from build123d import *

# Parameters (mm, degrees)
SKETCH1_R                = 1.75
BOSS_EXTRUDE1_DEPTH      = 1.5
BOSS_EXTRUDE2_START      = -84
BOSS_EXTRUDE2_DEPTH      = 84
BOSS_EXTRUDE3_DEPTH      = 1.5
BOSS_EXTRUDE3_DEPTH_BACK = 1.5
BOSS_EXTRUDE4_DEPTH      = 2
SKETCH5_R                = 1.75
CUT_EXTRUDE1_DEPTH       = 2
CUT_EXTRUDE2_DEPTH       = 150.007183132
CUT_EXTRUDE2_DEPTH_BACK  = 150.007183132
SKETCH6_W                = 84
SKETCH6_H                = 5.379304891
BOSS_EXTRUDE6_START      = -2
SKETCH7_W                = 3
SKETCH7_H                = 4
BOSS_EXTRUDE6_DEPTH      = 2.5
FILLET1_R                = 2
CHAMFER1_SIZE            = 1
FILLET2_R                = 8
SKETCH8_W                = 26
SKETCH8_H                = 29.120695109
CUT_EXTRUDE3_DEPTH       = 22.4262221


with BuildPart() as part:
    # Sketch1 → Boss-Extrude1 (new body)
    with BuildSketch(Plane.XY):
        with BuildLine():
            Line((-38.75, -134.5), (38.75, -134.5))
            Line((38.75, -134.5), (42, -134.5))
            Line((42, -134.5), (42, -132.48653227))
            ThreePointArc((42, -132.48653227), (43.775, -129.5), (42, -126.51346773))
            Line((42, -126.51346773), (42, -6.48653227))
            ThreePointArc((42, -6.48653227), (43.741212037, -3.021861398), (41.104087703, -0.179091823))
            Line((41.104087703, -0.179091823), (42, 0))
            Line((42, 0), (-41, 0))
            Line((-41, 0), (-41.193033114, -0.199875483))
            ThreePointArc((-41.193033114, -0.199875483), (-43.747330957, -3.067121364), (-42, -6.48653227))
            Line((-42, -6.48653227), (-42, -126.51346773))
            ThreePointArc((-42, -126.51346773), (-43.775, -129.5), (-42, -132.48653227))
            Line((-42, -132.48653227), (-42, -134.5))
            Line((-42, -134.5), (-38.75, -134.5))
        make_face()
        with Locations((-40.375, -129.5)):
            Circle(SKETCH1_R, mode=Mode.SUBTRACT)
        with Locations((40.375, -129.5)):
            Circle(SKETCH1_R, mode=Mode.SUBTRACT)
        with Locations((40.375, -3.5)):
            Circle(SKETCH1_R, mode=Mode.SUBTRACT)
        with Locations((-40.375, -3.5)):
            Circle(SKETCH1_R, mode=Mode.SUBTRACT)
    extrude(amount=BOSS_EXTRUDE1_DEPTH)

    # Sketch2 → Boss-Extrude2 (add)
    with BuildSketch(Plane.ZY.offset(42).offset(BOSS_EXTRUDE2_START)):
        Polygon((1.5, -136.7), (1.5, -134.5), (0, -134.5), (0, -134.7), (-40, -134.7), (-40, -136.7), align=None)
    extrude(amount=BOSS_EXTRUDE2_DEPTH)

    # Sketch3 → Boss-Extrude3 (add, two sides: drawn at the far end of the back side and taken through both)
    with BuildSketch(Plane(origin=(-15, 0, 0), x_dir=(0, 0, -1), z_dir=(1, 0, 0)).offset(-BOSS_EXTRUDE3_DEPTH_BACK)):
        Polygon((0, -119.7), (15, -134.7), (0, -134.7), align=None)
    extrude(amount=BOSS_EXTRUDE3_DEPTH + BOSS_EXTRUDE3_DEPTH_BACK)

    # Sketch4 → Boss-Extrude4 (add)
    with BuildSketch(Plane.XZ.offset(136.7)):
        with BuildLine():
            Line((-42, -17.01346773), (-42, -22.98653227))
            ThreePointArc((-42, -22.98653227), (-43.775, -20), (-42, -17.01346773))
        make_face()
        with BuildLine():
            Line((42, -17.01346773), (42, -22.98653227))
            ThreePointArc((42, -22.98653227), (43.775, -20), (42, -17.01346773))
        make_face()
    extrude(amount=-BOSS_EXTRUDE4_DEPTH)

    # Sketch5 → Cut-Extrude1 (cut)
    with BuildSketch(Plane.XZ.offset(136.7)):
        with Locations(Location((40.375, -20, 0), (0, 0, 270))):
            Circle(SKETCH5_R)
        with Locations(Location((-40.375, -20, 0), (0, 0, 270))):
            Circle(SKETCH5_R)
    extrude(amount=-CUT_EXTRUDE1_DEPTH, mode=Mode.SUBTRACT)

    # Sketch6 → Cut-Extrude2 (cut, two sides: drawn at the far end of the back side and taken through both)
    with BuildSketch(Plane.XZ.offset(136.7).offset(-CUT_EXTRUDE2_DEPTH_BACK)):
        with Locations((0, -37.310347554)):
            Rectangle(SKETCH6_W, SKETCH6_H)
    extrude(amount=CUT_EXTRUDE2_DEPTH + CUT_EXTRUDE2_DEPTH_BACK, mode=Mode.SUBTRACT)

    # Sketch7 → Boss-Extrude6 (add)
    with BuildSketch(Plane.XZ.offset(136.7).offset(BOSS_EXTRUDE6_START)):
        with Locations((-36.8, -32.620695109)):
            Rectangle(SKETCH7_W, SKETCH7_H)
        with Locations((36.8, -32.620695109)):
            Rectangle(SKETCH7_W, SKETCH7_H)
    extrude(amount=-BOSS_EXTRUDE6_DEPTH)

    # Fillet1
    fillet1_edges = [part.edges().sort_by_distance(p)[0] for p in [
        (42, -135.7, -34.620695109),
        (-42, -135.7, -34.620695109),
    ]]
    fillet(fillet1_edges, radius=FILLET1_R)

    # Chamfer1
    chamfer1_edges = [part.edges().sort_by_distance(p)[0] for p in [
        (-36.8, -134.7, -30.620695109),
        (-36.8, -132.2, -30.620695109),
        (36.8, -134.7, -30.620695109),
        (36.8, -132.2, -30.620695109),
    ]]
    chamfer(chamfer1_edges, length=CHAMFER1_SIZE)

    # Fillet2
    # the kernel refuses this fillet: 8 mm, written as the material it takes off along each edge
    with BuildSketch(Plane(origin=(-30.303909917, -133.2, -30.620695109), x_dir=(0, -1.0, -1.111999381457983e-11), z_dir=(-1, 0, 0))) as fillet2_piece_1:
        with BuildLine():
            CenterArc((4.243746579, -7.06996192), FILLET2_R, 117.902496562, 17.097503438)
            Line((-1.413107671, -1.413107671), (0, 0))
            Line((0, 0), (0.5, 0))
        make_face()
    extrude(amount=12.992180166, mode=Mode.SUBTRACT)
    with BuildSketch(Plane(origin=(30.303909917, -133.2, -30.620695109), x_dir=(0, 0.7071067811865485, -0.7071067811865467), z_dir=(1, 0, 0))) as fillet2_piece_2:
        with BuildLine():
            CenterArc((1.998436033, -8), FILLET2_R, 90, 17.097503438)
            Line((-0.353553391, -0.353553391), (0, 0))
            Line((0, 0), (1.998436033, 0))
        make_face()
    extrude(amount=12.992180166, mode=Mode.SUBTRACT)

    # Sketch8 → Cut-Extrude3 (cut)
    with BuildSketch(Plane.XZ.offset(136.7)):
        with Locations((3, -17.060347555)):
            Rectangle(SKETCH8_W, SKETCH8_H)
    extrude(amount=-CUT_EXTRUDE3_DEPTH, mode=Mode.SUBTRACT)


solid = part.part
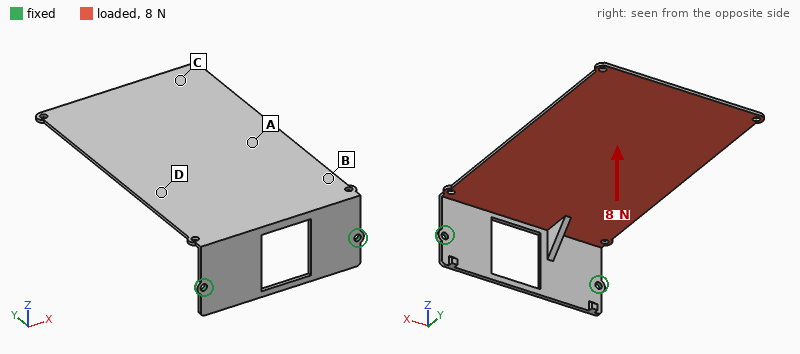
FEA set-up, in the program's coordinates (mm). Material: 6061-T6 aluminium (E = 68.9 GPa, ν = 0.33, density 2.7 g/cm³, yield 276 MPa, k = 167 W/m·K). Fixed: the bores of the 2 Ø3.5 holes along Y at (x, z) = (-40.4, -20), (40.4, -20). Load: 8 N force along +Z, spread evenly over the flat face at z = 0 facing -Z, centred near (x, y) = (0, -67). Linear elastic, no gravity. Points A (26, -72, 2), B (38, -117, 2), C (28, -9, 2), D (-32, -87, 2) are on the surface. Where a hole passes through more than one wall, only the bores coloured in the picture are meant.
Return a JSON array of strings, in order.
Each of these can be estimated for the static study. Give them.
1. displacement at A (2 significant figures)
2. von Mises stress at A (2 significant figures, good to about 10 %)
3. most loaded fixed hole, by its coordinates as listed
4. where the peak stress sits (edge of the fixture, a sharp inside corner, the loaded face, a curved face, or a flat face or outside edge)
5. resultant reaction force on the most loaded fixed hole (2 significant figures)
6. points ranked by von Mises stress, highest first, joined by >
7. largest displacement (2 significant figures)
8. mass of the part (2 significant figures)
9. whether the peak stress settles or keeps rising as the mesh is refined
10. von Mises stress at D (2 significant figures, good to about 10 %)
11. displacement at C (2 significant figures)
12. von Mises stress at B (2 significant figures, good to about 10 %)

["0.62 mm", "4.7 MPa", "(-40.4, -20)", "edge of the fixture", "5.5 N", "B > D > A > C", "1.8 mm", "59 g", "keeps rising", "7.6 MPa", "1.6 mm", "10 MPa"]
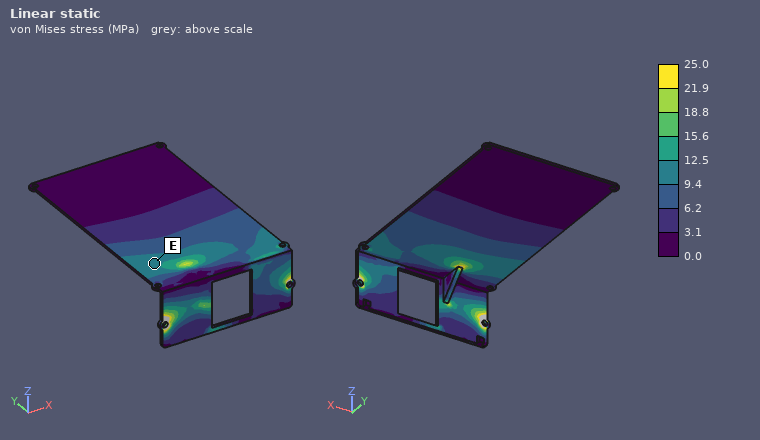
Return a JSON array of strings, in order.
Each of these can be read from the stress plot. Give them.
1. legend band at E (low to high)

["9.4 to 12.5 MPa"]
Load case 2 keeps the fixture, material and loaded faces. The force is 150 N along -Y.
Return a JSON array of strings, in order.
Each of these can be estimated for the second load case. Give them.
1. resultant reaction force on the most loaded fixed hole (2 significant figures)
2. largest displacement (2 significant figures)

["76 N", "1.6 mm"]
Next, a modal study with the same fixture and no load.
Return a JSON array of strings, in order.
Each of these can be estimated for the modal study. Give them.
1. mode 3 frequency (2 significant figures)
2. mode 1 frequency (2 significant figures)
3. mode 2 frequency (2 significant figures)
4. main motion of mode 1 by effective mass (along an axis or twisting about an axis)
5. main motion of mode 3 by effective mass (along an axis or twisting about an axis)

["320 Hz", "63 Hz", "230 Hz", "along Z", "along X"]
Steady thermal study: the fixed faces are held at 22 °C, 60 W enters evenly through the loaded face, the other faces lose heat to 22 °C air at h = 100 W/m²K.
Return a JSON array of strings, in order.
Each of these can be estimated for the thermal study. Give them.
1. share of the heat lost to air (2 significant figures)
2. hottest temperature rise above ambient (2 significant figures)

["85 %", "46 K"]
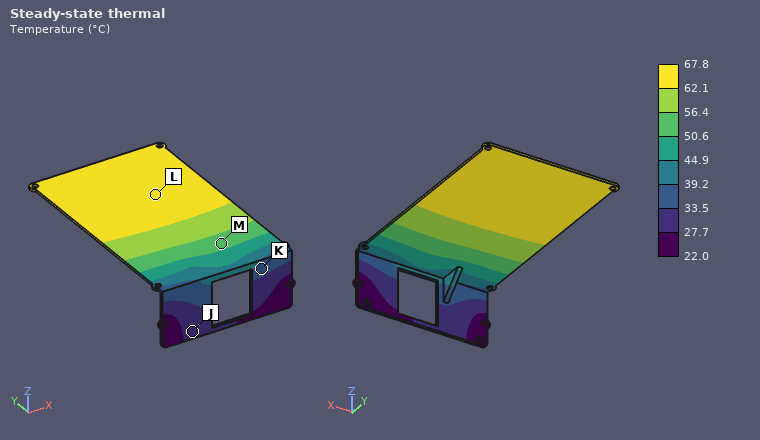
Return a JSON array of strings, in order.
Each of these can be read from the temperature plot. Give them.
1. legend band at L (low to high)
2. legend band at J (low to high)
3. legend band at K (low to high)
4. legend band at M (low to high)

["62.1 to 67.8 °C", "27.7 to 33.5 °C", "33.5 to 39.2 °C", "50.6 to 56.4 °C"]
